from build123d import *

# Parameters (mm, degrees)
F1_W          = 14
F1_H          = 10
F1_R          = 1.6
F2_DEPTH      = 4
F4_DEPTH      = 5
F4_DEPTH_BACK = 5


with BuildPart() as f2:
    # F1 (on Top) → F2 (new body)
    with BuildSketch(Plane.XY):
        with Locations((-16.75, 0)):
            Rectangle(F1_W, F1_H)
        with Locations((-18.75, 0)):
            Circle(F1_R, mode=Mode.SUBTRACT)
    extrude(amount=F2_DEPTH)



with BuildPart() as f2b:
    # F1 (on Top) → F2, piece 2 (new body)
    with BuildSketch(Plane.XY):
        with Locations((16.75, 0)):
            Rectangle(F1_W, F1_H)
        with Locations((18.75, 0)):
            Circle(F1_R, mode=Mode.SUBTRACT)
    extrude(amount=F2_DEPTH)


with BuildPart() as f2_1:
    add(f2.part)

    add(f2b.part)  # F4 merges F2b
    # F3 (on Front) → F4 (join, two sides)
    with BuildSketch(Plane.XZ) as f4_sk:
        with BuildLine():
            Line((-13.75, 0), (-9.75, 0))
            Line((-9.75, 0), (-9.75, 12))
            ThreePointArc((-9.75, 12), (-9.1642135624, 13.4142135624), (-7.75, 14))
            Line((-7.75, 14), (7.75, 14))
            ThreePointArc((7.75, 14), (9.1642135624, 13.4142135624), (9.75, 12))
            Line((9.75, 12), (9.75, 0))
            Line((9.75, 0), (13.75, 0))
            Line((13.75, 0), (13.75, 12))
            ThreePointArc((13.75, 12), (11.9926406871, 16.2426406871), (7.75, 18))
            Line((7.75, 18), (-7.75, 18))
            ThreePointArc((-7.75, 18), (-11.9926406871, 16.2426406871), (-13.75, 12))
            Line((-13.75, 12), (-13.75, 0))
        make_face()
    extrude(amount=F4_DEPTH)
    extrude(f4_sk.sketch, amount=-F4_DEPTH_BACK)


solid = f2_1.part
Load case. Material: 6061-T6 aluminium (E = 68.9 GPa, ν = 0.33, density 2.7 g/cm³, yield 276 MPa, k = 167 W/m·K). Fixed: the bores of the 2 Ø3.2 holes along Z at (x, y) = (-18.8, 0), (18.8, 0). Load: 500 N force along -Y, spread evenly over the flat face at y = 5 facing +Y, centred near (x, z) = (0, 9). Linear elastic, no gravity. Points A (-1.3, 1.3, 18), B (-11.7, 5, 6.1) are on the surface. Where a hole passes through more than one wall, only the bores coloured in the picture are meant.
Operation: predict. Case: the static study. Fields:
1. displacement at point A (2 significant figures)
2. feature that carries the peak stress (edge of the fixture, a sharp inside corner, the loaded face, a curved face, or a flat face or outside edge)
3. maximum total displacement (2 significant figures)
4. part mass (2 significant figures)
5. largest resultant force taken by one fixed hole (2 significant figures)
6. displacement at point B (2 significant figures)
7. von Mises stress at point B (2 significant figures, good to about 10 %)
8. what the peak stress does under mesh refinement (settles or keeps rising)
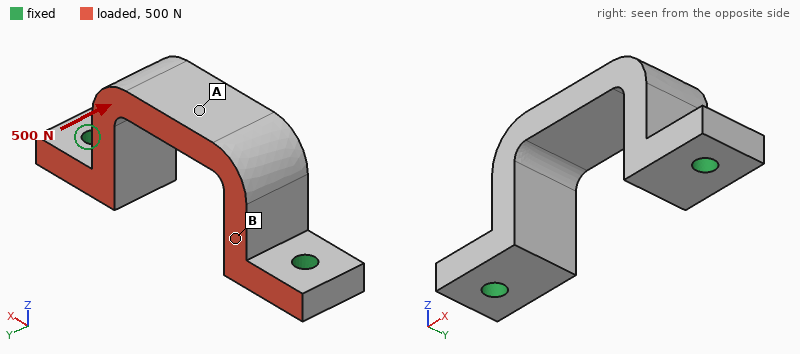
39 µm
edge of the fixture
41 µm
7.6 g
250 N
15 µm
16 MPa
keeps rising
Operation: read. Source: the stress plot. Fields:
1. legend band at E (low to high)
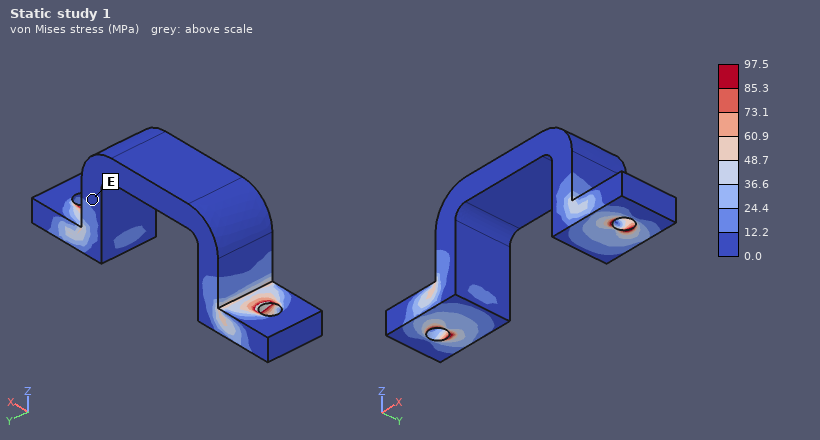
0.0 to 12.2 MPa
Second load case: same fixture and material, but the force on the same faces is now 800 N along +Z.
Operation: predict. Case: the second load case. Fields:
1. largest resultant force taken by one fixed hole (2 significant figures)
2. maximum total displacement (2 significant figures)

410 N
41 µm
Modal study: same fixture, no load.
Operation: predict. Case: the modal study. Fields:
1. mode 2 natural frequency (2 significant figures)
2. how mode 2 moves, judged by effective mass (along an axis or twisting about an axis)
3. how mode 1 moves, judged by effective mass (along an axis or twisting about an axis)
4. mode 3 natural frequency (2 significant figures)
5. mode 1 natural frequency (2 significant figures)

11 kHz
along X
along Y
15 kHz
7200 Hz
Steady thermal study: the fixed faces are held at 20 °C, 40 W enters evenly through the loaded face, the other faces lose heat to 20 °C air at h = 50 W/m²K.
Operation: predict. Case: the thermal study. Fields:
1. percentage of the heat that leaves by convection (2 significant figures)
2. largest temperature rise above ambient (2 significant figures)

4.1 %
36 K
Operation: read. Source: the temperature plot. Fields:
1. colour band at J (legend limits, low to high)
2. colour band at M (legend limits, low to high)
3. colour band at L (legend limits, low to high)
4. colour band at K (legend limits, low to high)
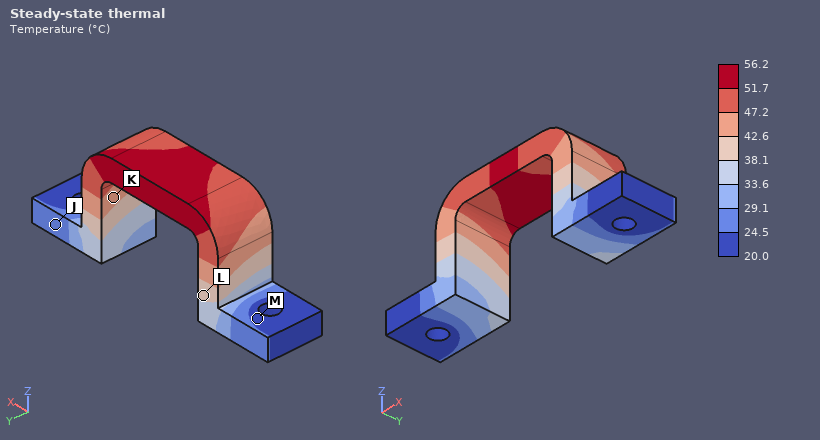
24.5 to 29.1 °C
20.0 to 24.5 °C
38.1 to 42.6 °C
42.6 to 47.2 °C
